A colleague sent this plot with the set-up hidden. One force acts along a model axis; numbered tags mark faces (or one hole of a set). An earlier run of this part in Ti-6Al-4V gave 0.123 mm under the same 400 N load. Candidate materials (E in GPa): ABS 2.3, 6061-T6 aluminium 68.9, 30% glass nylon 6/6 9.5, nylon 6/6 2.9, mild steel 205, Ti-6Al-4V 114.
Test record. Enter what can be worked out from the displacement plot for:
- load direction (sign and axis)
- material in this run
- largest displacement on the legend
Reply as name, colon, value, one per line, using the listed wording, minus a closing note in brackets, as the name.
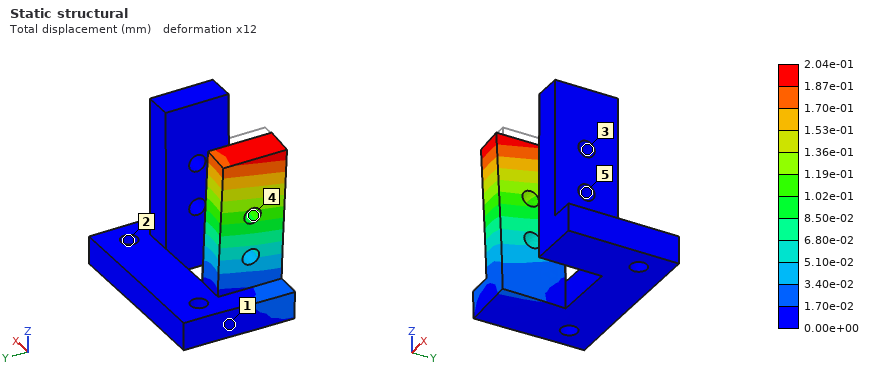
load direction: -X
material in this run: 6061-T6 aluminium
largest displacement on the legend: 2.04e-01 mm
